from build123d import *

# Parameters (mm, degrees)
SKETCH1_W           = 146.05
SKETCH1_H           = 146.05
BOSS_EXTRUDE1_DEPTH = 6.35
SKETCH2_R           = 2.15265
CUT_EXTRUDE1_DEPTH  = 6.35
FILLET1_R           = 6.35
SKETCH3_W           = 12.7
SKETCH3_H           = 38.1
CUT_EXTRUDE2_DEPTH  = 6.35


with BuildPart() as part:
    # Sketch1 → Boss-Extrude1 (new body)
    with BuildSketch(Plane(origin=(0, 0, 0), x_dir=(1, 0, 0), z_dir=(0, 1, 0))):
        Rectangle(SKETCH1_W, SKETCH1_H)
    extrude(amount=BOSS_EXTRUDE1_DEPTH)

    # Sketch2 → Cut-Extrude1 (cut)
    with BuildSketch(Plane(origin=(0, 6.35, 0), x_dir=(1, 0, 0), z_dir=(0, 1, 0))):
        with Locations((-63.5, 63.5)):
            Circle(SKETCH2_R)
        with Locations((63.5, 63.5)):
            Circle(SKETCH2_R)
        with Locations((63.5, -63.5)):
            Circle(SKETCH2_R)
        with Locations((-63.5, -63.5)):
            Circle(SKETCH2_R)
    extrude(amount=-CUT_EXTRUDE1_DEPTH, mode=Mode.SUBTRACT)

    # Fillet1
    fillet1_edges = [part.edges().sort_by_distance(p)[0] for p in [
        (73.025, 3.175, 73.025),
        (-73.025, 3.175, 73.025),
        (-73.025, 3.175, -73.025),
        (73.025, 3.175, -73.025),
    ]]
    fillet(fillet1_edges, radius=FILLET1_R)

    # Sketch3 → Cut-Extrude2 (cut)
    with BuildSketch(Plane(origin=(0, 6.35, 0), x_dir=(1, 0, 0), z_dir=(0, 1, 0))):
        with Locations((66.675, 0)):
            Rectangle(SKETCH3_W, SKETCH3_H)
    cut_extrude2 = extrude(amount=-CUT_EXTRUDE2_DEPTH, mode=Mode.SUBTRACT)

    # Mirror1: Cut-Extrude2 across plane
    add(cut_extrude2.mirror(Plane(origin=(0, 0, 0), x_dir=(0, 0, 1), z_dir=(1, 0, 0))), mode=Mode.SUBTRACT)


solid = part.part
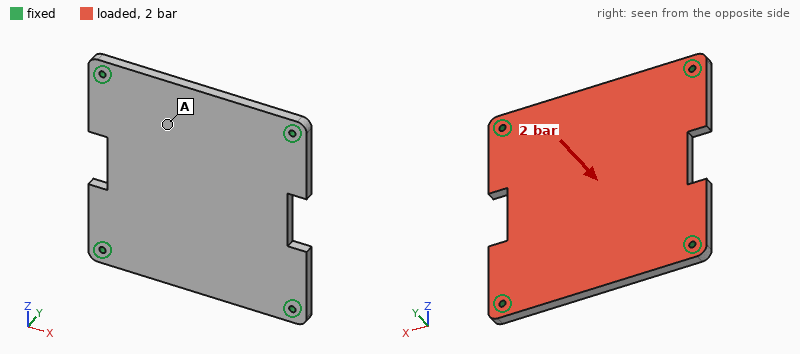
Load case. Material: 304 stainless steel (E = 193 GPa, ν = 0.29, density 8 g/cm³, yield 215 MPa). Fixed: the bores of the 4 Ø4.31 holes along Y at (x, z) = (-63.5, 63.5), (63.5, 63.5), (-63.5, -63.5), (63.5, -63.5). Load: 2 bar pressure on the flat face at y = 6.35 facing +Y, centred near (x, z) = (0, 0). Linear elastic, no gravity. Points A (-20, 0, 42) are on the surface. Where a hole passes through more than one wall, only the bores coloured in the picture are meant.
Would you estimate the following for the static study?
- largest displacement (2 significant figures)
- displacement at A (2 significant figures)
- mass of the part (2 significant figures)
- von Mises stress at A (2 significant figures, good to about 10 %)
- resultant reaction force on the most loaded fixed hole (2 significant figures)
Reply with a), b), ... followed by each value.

a) 0.11 mm
b) 0.074 mm
c) 1.0 kg
d) 22 MPa
e) 1.0 kN
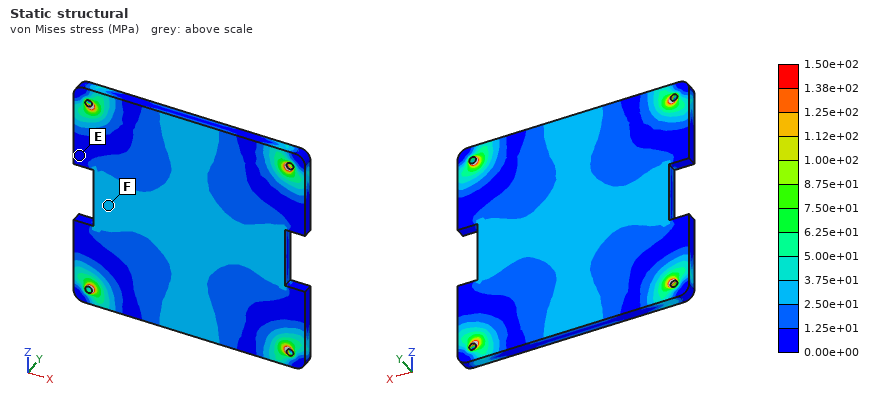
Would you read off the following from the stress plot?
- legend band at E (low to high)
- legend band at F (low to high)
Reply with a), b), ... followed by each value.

a) 0.00e+00 to 1.25e+01 MPa
b) 2.50e+01 to 3.75e+01 MPa
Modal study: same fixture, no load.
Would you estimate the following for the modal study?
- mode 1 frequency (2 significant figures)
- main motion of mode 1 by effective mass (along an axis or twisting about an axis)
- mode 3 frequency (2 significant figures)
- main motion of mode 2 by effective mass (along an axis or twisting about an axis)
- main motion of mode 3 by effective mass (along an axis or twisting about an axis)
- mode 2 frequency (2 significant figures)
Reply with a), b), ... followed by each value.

a) 1200 Hz
b) along Y
c) 2200 Hz
d) twisting about X
e) twisting about Z
f) 2000 Hz
